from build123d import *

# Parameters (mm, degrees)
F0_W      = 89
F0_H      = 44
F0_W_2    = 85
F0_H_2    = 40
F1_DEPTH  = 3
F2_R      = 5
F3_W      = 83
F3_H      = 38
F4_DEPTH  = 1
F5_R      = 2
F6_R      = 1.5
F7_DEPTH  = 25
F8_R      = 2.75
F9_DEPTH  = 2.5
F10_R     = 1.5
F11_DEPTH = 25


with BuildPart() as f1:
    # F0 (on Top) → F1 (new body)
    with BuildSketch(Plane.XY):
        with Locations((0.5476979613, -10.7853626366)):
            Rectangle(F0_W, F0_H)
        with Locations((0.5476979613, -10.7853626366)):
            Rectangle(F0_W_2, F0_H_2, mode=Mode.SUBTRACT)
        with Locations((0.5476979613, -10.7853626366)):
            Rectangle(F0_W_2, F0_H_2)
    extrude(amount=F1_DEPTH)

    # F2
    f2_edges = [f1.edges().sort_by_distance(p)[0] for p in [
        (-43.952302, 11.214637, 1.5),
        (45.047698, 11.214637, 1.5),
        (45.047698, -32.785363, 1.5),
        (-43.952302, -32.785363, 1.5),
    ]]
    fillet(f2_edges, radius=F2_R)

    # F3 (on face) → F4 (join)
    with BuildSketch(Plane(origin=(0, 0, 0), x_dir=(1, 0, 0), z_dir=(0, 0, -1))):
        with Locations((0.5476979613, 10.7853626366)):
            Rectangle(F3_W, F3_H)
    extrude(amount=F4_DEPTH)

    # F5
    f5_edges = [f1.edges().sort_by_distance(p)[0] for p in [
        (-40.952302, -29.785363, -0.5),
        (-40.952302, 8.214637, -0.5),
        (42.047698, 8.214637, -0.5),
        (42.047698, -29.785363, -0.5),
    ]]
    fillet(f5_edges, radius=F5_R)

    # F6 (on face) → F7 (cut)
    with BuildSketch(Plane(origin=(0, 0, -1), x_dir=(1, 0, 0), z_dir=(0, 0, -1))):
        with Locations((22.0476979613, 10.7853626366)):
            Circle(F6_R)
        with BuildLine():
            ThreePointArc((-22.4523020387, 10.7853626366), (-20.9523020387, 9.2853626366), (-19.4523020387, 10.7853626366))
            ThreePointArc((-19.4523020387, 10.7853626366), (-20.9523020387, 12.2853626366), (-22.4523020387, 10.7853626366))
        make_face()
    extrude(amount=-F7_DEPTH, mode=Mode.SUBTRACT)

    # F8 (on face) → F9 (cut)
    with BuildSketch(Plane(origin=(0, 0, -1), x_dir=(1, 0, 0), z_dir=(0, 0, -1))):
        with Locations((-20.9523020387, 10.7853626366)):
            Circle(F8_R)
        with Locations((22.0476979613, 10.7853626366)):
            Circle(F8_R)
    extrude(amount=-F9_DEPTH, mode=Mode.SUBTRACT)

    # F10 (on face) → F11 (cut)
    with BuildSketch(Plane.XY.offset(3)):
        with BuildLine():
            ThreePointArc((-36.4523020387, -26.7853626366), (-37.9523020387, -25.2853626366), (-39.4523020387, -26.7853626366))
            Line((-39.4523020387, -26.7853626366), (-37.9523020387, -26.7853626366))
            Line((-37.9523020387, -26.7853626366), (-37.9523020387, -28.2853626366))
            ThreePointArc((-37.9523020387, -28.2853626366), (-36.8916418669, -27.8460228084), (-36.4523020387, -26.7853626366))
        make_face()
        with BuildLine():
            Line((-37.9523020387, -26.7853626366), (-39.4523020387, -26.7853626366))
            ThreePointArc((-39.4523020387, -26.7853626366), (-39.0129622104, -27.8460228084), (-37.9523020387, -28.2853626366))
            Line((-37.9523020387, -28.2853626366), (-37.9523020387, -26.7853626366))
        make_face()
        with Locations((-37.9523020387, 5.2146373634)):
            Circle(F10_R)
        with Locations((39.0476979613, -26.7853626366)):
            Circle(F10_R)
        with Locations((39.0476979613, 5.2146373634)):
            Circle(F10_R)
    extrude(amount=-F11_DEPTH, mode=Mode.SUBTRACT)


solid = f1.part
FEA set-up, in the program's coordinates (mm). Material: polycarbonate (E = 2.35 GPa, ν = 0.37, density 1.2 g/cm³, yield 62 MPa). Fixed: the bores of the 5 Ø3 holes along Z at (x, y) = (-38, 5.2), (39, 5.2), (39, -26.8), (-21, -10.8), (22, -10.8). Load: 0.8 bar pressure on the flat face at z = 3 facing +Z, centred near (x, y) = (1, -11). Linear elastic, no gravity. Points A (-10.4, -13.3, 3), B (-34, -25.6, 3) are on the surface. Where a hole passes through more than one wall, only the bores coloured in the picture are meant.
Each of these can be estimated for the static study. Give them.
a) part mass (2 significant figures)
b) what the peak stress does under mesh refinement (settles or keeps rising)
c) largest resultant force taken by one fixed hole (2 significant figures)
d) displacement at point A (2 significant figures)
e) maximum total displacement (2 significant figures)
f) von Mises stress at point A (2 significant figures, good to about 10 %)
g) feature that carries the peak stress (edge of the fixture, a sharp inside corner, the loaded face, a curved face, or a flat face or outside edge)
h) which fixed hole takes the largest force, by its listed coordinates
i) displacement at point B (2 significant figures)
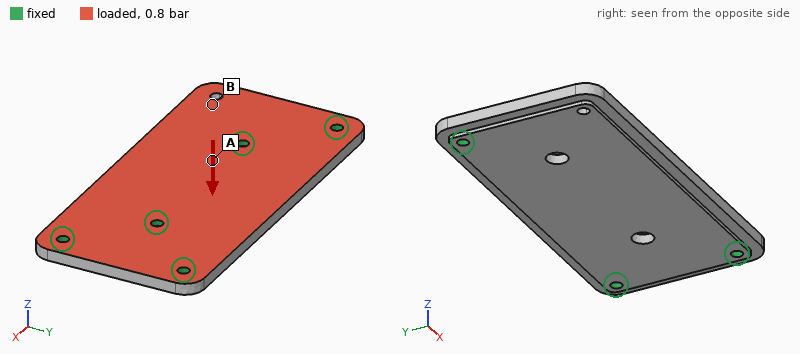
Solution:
17 g
keeps rising
140 N
0.11 mm
0.45 mm
4.5 MPa
edge of the fixture
(-21, -10.8)
0.29 mm
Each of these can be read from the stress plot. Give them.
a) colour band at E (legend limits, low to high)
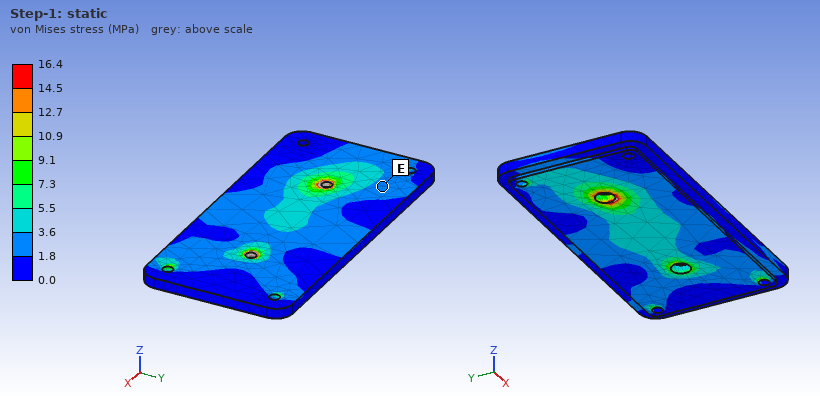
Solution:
1.8 to 3.6 MPa
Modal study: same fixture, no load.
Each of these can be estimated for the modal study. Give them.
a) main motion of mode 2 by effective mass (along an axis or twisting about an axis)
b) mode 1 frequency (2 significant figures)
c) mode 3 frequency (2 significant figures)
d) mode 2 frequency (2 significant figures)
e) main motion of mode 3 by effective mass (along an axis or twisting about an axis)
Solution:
along Z
1100 Hz
1700 Hz
1600 Hz
along Z
